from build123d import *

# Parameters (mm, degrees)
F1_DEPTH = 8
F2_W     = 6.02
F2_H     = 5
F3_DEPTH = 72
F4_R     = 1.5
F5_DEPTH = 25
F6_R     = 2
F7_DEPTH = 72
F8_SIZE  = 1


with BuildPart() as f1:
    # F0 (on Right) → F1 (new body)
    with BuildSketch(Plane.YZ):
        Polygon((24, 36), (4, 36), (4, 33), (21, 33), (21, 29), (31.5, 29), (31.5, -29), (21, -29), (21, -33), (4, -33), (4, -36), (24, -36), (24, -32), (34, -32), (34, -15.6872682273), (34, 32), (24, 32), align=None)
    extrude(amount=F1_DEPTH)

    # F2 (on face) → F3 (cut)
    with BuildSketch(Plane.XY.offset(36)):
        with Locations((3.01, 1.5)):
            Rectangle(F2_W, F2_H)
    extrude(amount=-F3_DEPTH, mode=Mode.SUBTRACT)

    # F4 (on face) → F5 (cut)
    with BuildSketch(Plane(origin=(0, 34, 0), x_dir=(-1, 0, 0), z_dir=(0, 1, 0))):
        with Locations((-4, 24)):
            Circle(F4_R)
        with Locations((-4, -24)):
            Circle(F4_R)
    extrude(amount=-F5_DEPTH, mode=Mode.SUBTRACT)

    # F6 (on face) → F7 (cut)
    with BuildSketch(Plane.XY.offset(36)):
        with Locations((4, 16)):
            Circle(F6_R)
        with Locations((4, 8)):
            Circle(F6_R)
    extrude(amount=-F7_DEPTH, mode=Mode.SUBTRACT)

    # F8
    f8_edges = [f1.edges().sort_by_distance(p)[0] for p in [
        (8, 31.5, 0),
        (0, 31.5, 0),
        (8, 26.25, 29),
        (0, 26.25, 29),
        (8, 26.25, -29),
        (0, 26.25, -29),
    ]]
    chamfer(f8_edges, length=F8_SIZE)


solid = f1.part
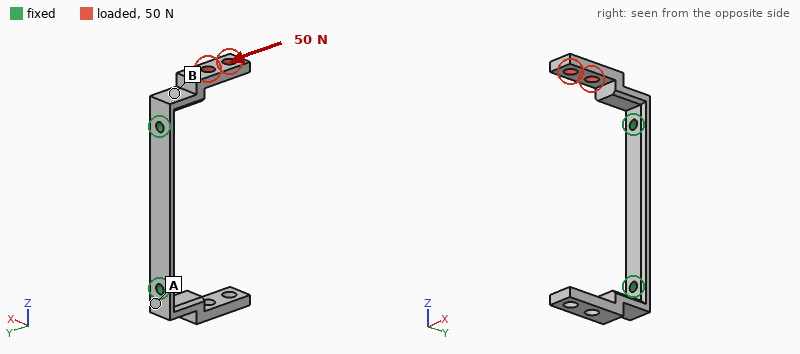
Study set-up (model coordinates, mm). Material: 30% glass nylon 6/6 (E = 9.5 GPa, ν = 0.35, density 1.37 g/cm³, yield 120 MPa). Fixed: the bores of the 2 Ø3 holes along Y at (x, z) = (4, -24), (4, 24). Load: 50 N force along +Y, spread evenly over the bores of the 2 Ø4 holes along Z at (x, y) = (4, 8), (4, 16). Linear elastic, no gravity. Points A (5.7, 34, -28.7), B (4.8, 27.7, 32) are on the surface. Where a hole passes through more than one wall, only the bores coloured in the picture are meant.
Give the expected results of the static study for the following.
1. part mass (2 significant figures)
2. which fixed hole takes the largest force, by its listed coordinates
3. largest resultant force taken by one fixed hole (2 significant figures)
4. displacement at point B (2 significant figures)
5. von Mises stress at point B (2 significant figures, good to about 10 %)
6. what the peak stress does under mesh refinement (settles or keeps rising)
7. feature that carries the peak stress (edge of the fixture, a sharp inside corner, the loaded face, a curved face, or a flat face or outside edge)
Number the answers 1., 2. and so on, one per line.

1. 3.5 g
2. (4, 24)
3. 50 N
4. 0.16 mm
5. 19 MPa
6. keeps rising
7. edge of the fixture
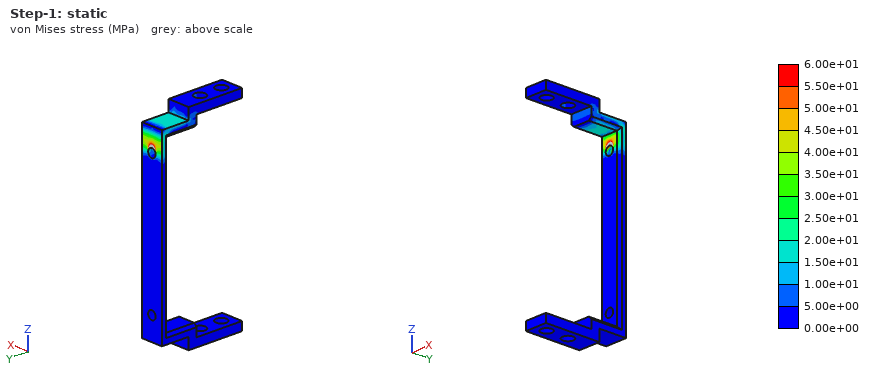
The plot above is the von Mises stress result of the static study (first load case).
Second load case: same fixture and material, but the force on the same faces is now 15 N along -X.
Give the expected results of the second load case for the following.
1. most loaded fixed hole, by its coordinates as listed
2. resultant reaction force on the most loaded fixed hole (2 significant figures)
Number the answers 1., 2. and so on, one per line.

1. (4, 24)
2. 16 N
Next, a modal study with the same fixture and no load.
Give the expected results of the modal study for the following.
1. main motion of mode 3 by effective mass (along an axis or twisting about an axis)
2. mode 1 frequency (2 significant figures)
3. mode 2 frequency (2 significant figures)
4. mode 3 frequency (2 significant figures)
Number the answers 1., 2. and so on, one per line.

1. along X
2. 1000 Hz
3. 1000 Hz
4. 1600 Hz
